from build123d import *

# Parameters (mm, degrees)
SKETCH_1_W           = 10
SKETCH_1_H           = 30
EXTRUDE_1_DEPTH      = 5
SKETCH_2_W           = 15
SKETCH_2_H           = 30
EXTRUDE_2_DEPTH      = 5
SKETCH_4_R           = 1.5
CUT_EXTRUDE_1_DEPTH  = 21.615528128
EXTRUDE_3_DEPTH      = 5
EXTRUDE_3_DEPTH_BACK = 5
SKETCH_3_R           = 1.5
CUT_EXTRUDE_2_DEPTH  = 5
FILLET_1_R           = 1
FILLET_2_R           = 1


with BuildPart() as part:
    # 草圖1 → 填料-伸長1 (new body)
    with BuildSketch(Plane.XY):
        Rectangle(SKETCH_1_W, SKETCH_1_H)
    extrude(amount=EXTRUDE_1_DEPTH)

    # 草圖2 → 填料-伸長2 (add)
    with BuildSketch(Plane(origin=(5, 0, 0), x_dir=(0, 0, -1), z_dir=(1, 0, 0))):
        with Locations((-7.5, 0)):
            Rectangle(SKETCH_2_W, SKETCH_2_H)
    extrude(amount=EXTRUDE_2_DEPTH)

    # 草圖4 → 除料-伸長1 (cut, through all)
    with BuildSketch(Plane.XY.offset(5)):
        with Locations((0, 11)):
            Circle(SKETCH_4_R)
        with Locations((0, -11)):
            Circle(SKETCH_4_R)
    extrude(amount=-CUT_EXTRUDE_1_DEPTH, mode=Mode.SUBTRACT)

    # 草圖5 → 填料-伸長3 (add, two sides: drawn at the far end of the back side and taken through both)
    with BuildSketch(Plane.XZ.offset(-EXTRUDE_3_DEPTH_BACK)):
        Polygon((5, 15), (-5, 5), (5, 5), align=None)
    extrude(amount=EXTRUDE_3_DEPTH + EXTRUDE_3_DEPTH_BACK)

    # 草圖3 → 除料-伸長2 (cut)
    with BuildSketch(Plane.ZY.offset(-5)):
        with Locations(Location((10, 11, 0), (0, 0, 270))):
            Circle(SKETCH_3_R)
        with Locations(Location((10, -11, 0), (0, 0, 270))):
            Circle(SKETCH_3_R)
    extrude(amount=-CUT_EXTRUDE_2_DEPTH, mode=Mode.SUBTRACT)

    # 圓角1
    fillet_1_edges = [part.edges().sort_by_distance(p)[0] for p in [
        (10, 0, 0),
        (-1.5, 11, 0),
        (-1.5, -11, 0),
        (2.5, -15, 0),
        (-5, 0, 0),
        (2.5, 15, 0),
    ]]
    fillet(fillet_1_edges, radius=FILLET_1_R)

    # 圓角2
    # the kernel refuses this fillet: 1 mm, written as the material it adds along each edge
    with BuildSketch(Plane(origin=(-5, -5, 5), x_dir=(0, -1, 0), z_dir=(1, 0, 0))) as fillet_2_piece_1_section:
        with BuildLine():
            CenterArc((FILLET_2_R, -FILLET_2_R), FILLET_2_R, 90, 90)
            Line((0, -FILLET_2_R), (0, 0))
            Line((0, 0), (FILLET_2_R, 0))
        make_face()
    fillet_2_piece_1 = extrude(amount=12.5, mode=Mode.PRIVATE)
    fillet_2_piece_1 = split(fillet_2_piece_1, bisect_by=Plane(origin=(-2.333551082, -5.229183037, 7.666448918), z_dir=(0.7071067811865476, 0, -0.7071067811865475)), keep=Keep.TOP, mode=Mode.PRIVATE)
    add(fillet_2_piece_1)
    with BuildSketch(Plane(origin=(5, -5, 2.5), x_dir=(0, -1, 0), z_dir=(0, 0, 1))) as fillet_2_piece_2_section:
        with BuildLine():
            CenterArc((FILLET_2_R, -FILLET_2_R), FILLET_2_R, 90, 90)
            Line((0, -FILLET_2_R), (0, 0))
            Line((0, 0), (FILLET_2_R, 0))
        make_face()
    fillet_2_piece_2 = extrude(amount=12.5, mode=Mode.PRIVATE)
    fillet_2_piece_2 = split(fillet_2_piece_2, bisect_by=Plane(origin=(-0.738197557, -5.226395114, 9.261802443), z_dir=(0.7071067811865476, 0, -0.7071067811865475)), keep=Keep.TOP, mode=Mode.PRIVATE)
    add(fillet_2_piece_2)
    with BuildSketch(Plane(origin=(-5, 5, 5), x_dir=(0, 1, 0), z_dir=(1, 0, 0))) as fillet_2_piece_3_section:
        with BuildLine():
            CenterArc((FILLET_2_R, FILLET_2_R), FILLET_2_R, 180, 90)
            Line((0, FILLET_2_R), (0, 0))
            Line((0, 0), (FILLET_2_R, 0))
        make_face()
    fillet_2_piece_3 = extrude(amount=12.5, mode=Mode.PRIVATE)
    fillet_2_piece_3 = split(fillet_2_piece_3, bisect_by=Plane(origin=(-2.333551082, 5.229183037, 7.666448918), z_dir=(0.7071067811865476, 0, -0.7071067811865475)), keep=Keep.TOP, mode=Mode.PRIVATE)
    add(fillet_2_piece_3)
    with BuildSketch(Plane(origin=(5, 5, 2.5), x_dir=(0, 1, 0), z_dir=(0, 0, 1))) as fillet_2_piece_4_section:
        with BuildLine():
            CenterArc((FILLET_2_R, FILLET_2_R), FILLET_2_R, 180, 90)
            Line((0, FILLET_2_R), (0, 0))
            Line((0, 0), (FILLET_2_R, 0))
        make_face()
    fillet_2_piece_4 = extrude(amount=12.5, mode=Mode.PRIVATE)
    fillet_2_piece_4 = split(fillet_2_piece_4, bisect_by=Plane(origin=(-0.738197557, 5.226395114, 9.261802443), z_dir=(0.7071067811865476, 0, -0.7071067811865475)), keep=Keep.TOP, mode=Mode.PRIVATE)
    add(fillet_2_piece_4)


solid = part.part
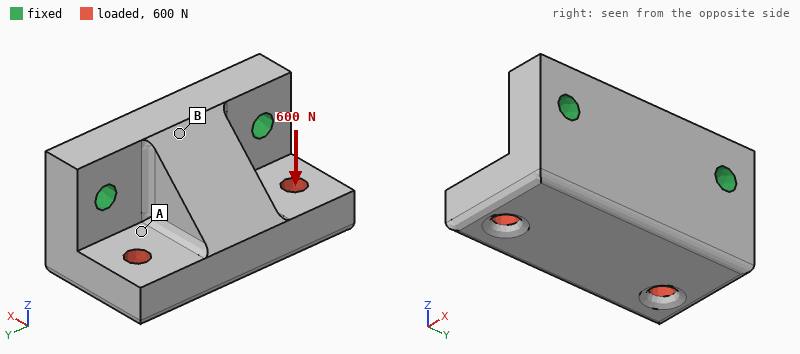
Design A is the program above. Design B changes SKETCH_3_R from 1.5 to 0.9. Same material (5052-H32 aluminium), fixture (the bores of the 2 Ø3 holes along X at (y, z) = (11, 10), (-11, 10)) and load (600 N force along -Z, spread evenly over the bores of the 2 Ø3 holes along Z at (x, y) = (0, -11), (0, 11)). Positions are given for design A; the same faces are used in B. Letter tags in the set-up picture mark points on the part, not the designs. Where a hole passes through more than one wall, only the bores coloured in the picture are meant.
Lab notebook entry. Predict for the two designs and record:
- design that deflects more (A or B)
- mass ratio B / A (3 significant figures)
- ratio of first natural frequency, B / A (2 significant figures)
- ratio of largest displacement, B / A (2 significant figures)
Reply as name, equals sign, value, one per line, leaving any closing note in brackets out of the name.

design that deflects more = B
mass ratio B / A = 1.01
ratio of first natural frequency, B / A = 0.85
ratio of largest displacement, B / A = 1.3
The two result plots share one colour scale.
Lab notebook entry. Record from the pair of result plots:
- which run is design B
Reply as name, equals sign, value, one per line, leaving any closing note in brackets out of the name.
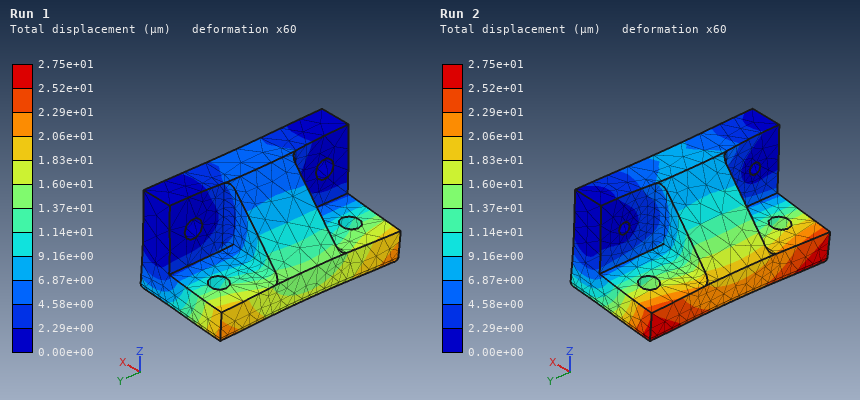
which run is design B = Run 2
